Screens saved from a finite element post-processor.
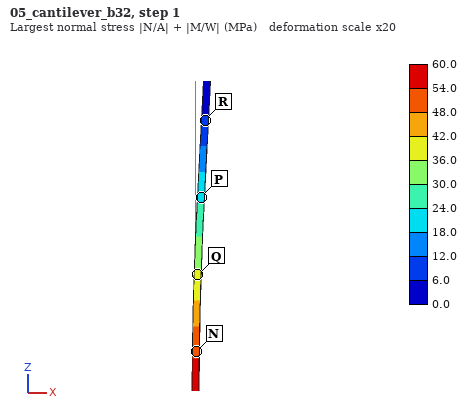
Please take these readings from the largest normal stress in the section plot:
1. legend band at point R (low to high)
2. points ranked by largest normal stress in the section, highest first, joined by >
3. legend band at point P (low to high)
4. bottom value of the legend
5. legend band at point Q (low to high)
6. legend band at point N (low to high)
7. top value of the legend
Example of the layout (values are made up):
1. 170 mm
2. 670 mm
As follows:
1. 6.0 to 12.0 MPa
2. N > Q > P > R
3. 18.0 to 24.0 MPa
4. 0.0 MPa
5. 36.0 to 42.0 MPa
6. 48.0 to 54.0 MPa
7. 60.0 MPa
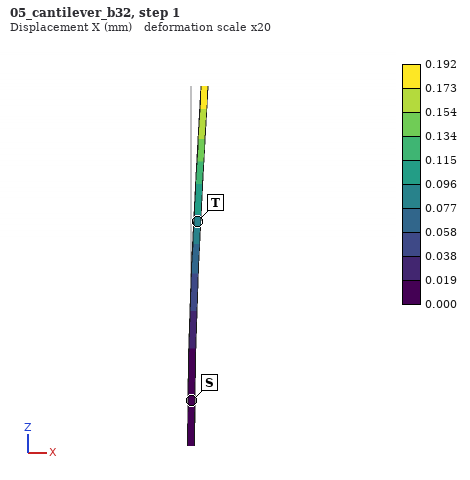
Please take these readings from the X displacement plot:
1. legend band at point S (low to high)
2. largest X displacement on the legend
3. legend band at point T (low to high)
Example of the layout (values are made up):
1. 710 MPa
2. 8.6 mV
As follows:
1. 0.000 to 0.019 mm
2. 0.192 mm
3. 0.077 to 0.096 mm
